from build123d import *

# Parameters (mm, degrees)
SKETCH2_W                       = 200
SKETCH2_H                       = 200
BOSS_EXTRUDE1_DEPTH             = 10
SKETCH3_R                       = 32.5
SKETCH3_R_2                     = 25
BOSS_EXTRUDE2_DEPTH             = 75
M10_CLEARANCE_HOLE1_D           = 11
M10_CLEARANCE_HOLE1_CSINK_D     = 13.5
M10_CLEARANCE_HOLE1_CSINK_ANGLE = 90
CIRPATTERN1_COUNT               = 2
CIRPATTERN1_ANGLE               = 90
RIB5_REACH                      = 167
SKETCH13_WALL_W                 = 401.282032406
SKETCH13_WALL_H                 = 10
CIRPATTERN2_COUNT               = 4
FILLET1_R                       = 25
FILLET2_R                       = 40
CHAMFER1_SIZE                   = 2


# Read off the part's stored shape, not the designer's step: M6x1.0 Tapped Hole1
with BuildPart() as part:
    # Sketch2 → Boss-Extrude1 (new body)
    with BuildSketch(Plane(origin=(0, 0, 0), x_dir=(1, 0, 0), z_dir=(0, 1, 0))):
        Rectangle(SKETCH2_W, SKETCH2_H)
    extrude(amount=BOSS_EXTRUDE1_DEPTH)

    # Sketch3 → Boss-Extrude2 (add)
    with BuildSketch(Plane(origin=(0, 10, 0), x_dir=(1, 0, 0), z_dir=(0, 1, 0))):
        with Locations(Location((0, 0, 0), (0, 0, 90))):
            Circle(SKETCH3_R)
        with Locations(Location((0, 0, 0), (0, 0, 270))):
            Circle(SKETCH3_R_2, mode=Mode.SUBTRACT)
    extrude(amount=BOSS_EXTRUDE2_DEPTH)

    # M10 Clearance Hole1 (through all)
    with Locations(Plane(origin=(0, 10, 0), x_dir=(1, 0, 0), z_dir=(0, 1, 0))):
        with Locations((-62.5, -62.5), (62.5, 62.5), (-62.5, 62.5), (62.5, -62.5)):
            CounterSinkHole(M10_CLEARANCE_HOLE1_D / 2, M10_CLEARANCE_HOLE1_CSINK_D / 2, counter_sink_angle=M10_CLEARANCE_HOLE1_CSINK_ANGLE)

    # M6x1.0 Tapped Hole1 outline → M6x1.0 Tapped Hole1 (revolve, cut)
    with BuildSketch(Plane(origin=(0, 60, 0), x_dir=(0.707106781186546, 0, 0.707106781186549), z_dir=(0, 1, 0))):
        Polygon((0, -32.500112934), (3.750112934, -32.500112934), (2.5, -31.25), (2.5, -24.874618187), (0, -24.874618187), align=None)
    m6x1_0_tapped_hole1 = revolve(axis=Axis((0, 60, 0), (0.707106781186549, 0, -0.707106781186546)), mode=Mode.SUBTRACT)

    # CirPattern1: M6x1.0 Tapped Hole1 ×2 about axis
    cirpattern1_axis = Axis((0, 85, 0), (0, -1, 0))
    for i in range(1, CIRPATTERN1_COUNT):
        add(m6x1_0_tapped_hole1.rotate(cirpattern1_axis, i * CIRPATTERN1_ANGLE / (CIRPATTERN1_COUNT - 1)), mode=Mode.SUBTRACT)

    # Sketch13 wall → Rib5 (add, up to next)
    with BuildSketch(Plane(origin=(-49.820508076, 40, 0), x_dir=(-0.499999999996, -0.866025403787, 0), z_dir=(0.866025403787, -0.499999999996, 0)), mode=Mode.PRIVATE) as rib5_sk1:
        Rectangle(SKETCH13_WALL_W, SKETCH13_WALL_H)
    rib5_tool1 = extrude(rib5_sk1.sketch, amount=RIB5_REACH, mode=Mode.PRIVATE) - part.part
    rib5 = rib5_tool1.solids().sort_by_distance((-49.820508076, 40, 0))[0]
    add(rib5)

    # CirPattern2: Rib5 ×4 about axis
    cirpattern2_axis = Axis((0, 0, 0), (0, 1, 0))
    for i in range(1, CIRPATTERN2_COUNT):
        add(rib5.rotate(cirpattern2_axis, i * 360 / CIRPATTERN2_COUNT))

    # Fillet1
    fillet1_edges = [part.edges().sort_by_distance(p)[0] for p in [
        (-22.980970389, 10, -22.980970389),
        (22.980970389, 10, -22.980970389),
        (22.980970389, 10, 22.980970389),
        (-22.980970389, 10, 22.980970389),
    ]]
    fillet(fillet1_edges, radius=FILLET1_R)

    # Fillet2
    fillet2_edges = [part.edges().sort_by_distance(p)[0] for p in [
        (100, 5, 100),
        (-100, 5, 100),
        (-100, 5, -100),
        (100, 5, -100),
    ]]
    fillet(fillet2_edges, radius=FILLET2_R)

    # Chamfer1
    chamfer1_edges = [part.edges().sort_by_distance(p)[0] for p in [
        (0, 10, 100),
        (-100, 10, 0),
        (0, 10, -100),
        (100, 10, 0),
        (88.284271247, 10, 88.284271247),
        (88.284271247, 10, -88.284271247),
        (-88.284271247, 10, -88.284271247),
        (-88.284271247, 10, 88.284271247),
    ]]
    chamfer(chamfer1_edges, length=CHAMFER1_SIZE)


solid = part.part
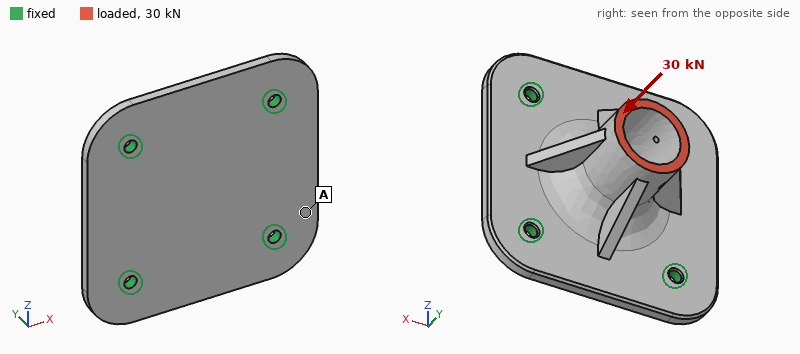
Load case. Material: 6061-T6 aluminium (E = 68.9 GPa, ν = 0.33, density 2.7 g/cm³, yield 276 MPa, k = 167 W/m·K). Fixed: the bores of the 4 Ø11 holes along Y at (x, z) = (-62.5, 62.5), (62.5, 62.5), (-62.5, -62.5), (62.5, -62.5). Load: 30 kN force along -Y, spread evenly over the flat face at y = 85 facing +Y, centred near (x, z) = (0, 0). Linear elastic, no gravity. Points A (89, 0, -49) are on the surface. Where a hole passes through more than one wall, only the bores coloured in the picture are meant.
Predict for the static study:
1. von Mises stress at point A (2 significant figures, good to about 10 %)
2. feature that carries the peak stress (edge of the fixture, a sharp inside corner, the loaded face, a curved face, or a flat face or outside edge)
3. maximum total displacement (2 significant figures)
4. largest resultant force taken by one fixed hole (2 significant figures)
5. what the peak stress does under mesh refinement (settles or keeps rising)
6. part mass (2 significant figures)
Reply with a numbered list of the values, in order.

1. 20 MPa
2. edge of the fixture
3. 0.20 mm
4. 8.4 kN
5. keeps rising
6. 1.5 kg
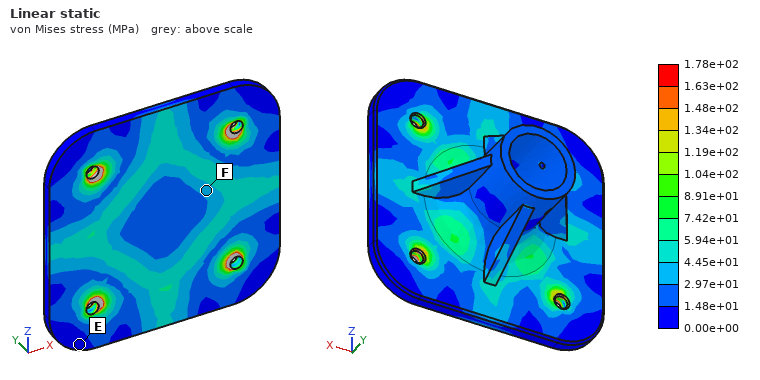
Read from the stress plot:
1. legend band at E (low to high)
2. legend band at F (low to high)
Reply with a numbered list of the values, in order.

1. 0.00e+00 to 1.48e+01 MPa
2. 2.97e+01 to 4.45e+01 MPa
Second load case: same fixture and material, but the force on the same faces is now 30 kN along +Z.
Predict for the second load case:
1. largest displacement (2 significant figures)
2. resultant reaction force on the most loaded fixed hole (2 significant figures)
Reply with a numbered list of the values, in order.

1. 0.62 mm
2. 13 kN
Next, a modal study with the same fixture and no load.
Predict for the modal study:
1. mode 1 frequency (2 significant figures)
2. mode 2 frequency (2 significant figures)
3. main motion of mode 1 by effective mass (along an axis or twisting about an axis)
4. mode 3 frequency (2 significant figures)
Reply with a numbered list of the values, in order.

1. 2100 Hz
2. 2400 Hz
3. along Y
4. 2400 Hz
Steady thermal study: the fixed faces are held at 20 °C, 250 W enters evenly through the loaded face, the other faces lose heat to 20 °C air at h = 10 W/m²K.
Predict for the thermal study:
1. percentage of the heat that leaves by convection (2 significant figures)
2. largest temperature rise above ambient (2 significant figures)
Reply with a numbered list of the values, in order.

1. 10 %
2. 85 K
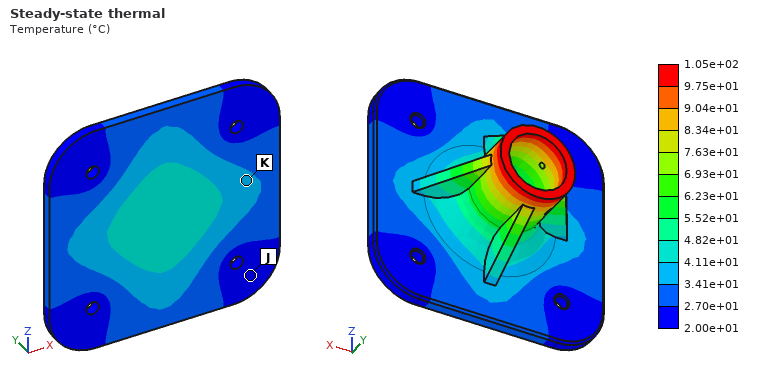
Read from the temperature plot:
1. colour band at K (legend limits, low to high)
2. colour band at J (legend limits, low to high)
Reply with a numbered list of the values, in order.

1. 3.41e+01 to 4.11e+01 °C
2. 2.00e+01 to 2.70e+01 °C
